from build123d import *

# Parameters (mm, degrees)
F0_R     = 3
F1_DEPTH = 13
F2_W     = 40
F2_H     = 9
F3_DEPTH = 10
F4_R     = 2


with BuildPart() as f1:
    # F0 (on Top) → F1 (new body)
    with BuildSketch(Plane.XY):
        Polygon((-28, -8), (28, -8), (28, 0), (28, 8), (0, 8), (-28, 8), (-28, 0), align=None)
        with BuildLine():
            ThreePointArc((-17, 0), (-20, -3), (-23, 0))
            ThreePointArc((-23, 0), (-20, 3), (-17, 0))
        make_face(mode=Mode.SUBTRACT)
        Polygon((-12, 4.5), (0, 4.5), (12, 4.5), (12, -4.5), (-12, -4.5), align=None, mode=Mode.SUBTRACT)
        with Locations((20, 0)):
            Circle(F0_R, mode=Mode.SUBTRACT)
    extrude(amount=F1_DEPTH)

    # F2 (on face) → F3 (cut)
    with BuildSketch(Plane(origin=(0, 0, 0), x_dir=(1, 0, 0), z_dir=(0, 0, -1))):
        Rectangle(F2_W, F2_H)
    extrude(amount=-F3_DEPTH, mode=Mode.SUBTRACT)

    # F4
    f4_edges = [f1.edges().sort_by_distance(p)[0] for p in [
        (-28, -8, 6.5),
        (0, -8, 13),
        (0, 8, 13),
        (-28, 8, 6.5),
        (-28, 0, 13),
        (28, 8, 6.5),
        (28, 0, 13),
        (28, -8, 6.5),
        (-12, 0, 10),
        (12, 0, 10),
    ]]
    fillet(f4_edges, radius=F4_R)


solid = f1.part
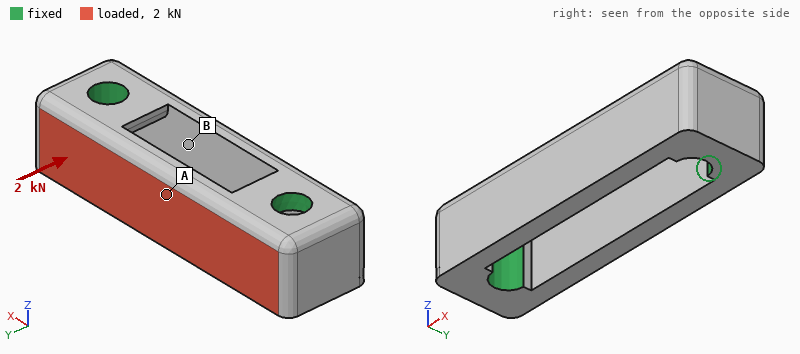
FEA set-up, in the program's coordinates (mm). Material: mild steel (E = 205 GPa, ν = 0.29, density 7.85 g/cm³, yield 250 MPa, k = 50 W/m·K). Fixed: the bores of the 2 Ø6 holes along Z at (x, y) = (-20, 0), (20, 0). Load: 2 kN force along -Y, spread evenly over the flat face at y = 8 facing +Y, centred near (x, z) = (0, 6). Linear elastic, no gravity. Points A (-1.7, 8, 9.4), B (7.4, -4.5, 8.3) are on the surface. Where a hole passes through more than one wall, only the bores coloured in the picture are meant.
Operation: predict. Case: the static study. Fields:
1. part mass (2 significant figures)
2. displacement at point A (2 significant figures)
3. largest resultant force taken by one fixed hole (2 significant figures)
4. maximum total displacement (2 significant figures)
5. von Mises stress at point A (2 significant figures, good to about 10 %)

53 g
17 µm
1.0 kN
32 µm
83 MPa
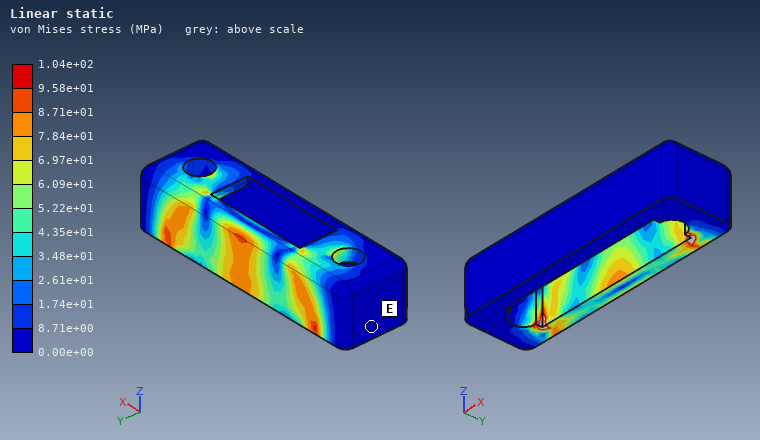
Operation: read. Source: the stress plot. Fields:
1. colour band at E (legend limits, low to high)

0.00e+00 to 8.71e+00 MPa
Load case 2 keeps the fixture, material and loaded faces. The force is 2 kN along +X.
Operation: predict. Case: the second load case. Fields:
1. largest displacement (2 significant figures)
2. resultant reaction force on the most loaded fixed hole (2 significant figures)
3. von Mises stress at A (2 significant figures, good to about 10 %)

1.9 µm
1.0 kN
7.8 MPa
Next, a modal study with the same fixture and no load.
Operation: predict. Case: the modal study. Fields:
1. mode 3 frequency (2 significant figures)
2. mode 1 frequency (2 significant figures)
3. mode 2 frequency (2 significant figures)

24 kHz
13 kHz
13 kHz
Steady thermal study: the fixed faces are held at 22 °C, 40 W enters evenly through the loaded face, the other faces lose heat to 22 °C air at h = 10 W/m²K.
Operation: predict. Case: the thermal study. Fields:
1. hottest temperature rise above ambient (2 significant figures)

76 K
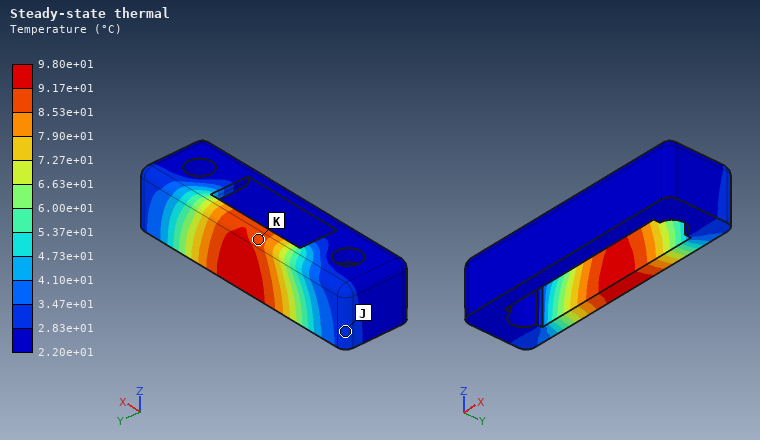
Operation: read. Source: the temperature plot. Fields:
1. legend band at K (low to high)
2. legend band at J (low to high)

8.53e+01 to 9.17e+01 °C
2.83e+01 to 3.47e+01 °C
